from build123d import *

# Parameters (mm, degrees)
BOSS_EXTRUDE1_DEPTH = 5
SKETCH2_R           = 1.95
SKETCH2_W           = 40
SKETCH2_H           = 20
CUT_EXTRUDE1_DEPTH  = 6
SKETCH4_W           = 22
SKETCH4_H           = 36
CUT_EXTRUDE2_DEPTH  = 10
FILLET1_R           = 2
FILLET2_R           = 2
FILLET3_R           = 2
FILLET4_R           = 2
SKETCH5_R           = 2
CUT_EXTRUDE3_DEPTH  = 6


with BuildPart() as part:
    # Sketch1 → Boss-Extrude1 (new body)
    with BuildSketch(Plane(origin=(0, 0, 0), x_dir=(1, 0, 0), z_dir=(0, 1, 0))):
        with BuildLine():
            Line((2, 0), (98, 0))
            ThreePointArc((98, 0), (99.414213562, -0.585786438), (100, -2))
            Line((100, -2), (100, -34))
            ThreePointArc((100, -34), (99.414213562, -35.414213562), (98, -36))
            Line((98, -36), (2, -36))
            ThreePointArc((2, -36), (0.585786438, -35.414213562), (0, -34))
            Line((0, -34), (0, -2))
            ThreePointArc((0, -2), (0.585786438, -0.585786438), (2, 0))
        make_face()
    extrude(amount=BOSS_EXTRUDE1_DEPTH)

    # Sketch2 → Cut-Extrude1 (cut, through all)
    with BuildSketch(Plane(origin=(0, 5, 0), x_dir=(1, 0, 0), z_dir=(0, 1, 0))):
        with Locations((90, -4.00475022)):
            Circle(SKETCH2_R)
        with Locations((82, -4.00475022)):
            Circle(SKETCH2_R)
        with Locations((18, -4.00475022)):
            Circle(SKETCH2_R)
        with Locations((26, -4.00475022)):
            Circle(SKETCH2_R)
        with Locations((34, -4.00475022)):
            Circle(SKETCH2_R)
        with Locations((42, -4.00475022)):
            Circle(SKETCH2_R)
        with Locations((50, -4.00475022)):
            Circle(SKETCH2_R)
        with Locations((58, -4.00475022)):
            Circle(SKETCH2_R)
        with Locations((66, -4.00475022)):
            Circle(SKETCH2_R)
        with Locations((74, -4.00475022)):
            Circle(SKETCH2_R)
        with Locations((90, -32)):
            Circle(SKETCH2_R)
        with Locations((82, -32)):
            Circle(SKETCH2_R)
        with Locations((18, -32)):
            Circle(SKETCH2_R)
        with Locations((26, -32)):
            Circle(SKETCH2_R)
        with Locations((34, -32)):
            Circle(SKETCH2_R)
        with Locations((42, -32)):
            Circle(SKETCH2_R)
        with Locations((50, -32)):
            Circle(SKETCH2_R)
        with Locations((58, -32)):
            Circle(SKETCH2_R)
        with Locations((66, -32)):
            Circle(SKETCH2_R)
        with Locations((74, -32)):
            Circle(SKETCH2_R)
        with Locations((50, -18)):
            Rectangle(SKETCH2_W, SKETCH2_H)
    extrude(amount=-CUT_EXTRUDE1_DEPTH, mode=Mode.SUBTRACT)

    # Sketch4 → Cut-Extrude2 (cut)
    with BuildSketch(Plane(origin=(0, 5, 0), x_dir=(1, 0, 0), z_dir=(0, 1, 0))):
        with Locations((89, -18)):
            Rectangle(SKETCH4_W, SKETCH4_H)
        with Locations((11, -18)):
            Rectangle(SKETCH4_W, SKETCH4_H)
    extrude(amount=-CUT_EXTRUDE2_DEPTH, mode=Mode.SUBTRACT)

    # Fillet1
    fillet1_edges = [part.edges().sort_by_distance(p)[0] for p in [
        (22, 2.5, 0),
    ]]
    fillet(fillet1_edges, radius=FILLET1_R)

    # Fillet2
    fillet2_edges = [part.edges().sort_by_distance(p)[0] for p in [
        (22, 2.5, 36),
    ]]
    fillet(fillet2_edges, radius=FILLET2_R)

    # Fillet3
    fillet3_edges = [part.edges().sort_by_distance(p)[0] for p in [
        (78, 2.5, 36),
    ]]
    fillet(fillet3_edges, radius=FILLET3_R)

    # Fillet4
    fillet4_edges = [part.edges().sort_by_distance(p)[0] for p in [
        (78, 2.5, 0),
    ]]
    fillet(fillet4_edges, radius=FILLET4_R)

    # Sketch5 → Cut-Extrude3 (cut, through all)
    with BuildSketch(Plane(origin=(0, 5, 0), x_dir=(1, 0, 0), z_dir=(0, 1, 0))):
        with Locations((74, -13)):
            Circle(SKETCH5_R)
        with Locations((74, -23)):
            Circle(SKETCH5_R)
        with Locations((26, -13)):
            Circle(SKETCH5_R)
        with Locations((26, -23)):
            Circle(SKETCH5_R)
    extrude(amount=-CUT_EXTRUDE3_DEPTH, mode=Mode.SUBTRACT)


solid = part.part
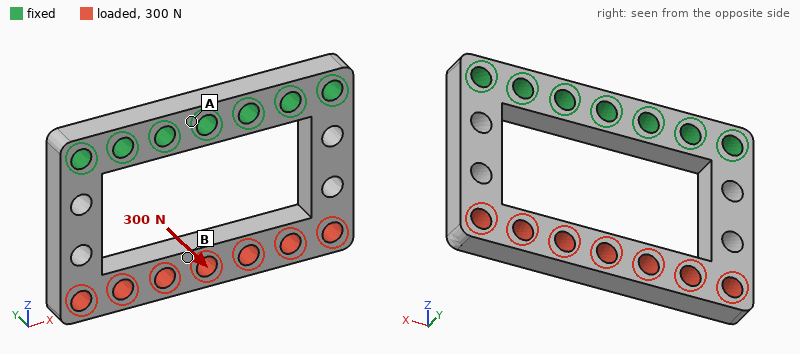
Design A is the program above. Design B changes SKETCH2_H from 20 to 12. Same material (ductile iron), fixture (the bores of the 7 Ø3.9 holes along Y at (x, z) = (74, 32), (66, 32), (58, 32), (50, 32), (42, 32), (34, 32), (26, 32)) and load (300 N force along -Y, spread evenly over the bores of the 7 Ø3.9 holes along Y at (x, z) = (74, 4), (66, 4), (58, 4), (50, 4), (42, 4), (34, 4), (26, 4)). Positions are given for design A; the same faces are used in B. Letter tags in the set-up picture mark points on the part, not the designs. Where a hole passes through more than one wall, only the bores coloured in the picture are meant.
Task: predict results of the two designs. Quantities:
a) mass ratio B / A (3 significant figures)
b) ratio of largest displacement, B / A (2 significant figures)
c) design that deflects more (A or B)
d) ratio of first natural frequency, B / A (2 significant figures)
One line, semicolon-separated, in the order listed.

1.32; 0.83; A; 0.99
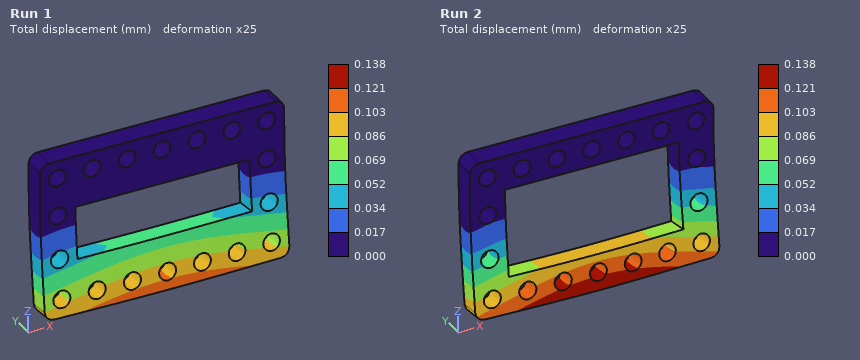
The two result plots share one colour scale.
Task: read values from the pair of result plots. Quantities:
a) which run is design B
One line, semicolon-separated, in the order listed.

Run 1
